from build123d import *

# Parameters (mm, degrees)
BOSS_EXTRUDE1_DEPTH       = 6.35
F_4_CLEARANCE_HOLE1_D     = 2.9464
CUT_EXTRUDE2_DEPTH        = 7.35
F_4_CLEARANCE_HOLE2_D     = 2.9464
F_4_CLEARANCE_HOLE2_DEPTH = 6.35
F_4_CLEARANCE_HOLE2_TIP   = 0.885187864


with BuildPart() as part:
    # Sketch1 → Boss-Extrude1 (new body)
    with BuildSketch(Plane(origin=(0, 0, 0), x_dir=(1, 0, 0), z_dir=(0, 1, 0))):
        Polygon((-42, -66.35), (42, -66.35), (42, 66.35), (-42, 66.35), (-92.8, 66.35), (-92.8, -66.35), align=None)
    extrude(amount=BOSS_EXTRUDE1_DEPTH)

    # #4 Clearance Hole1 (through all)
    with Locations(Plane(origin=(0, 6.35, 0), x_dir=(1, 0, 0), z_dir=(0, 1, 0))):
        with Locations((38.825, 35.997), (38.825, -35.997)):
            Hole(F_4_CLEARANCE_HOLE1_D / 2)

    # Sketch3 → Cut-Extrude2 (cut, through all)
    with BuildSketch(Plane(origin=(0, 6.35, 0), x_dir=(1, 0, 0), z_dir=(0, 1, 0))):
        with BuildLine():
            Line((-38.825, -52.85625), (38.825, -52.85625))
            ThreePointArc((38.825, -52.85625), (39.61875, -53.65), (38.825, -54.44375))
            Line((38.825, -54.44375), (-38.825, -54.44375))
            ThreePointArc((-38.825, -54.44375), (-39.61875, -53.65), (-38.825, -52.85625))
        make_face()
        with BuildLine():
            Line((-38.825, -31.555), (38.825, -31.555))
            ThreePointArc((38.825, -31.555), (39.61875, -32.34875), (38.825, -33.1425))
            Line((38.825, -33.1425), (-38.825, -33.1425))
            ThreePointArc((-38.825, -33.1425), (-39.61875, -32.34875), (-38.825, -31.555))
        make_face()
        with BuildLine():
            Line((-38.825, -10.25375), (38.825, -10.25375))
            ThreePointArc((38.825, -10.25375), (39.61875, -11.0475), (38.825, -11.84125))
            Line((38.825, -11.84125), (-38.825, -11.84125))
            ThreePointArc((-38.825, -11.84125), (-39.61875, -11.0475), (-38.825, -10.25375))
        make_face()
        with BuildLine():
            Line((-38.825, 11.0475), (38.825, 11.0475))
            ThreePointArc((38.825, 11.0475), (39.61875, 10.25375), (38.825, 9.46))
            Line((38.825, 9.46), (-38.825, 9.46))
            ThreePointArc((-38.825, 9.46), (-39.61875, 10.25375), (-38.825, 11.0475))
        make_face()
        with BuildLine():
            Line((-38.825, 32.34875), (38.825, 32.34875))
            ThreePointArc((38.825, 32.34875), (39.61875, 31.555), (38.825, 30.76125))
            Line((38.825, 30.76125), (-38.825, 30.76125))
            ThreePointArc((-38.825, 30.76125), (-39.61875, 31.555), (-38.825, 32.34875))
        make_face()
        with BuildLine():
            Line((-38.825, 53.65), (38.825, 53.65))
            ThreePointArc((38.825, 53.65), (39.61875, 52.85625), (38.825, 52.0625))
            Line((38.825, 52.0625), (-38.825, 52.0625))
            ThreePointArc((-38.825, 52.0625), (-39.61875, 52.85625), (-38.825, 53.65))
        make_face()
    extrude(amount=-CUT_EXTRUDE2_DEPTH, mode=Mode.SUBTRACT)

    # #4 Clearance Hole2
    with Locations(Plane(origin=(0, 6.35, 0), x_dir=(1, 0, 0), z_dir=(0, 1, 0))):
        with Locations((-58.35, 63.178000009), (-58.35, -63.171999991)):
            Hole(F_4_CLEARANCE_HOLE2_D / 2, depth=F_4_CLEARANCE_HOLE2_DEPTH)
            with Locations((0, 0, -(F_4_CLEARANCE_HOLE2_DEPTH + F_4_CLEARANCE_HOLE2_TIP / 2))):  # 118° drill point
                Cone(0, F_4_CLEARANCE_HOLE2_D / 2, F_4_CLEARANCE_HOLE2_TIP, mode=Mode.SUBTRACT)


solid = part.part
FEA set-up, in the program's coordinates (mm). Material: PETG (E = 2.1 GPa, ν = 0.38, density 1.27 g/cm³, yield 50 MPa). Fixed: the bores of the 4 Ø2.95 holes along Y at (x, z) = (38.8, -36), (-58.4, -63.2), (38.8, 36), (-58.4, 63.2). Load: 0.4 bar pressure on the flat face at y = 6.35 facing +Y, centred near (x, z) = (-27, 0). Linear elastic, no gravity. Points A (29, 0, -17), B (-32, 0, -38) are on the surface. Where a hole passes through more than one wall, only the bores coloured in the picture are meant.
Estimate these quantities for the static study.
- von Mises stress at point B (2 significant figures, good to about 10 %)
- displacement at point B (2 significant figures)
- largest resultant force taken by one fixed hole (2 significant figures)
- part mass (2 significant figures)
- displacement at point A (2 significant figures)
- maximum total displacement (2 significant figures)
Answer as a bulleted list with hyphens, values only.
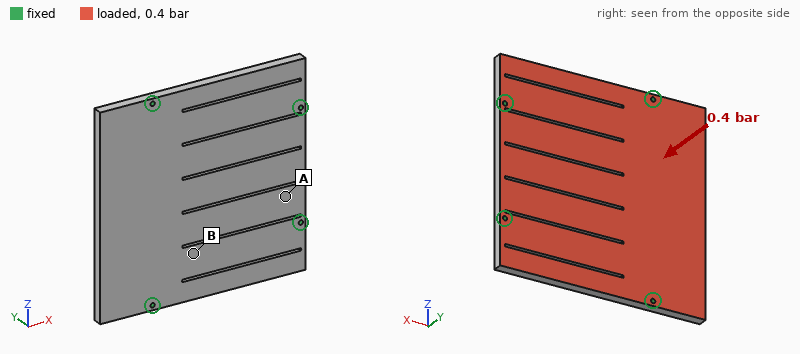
- 4.1 MPa
- 0.79 mm
- 220 N
- 140 g
- 0.70 mm
- 1.6 mm
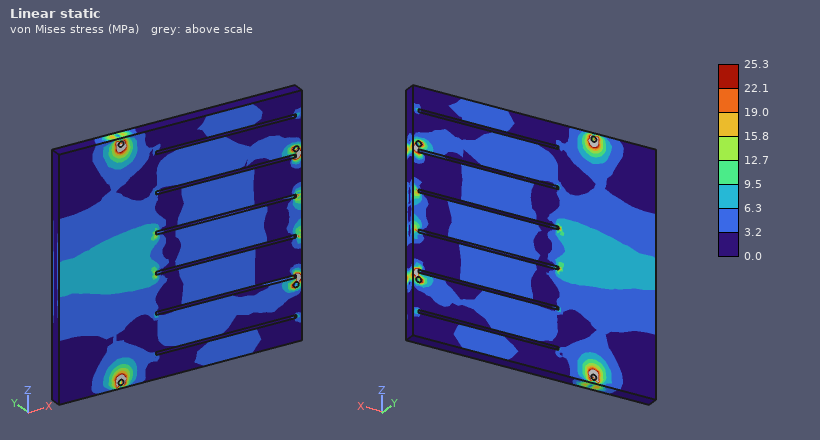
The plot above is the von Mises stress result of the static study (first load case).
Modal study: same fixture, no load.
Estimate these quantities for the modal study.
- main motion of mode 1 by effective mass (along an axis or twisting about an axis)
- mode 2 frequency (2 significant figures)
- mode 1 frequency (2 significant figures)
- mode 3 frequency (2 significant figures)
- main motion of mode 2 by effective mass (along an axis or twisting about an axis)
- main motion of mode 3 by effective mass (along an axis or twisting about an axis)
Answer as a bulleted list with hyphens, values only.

- along Y
- 430 Hz
- 330 Hz
- 580 Hz
- twisting about Z
- twisting about X
